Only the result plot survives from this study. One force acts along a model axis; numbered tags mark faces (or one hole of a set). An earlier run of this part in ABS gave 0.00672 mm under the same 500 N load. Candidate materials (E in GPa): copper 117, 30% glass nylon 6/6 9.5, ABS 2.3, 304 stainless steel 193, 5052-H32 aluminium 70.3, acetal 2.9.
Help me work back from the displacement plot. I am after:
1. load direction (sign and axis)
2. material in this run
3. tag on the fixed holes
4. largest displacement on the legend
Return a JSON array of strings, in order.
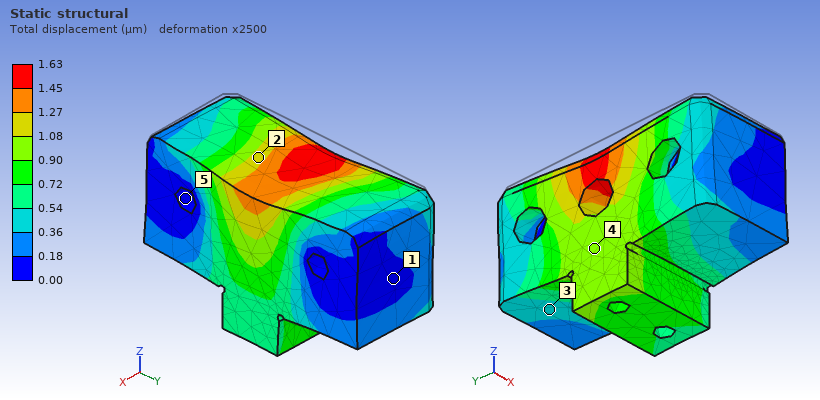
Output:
["-Z", "30% glass nylon 6/6", "5", "1.63 µm"]
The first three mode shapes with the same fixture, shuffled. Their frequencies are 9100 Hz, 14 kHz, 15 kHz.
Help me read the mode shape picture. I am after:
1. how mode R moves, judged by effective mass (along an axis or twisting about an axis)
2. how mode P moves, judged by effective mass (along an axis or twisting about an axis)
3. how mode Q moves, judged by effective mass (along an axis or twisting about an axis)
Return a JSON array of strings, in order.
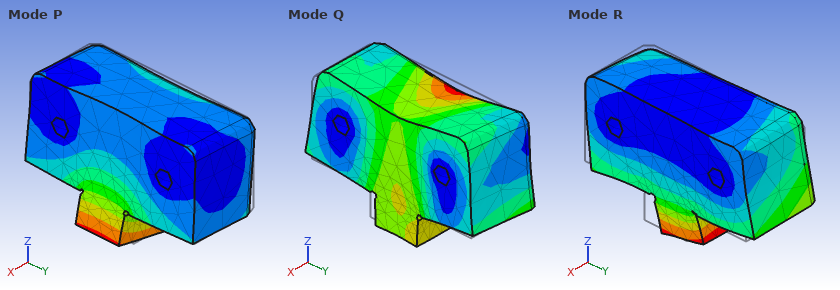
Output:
["along Y", "along X", "along Z"]
